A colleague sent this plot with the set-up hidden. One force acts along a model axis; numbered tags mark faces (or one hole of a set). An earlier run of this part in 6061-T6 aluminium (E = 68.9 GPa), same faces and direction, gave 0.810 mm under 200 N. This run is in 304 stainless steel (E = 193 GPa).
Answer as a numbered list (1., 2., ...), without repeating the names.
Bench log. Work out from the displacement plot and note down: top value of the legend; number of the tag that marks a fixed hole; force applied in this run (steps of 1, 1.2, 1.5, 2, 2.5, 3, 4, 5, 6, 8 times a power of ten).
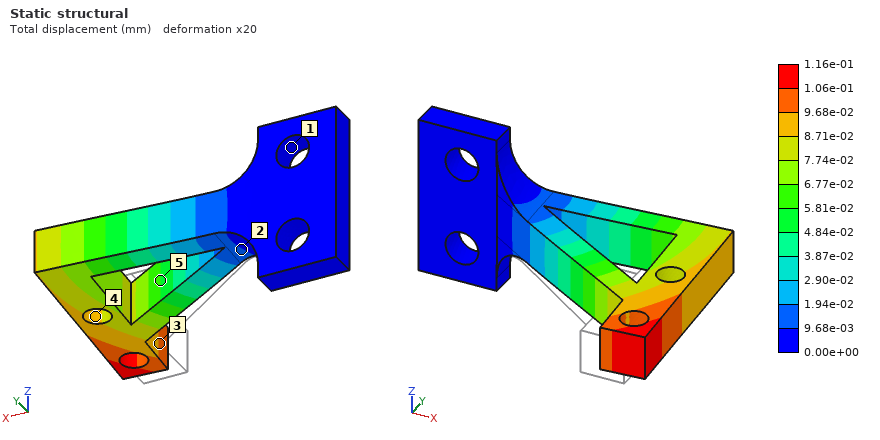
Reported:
1. 1.16e-01 mm
2. 1
3. 80 N
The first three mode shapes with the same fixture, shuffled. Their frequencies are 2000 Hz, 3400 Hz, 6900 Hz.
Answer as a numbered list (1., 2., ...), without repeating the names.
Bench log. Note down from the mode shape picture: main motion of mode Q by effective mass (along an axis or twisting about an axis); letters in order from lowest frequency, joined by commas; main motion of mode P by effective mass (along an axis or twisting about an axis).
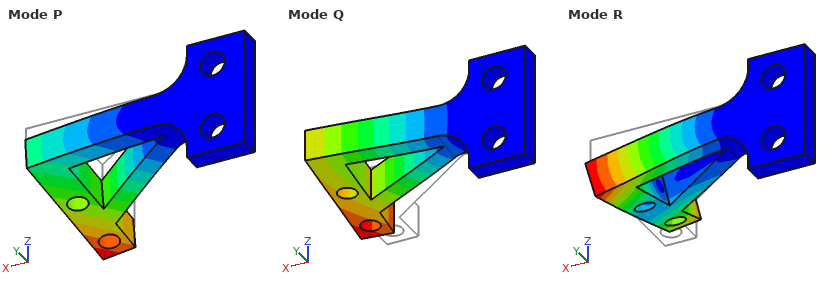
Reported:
1. along Y
2. Q, P, R
3. along Z
